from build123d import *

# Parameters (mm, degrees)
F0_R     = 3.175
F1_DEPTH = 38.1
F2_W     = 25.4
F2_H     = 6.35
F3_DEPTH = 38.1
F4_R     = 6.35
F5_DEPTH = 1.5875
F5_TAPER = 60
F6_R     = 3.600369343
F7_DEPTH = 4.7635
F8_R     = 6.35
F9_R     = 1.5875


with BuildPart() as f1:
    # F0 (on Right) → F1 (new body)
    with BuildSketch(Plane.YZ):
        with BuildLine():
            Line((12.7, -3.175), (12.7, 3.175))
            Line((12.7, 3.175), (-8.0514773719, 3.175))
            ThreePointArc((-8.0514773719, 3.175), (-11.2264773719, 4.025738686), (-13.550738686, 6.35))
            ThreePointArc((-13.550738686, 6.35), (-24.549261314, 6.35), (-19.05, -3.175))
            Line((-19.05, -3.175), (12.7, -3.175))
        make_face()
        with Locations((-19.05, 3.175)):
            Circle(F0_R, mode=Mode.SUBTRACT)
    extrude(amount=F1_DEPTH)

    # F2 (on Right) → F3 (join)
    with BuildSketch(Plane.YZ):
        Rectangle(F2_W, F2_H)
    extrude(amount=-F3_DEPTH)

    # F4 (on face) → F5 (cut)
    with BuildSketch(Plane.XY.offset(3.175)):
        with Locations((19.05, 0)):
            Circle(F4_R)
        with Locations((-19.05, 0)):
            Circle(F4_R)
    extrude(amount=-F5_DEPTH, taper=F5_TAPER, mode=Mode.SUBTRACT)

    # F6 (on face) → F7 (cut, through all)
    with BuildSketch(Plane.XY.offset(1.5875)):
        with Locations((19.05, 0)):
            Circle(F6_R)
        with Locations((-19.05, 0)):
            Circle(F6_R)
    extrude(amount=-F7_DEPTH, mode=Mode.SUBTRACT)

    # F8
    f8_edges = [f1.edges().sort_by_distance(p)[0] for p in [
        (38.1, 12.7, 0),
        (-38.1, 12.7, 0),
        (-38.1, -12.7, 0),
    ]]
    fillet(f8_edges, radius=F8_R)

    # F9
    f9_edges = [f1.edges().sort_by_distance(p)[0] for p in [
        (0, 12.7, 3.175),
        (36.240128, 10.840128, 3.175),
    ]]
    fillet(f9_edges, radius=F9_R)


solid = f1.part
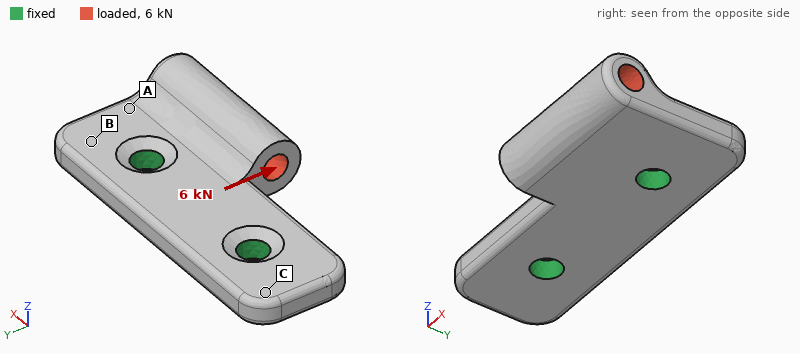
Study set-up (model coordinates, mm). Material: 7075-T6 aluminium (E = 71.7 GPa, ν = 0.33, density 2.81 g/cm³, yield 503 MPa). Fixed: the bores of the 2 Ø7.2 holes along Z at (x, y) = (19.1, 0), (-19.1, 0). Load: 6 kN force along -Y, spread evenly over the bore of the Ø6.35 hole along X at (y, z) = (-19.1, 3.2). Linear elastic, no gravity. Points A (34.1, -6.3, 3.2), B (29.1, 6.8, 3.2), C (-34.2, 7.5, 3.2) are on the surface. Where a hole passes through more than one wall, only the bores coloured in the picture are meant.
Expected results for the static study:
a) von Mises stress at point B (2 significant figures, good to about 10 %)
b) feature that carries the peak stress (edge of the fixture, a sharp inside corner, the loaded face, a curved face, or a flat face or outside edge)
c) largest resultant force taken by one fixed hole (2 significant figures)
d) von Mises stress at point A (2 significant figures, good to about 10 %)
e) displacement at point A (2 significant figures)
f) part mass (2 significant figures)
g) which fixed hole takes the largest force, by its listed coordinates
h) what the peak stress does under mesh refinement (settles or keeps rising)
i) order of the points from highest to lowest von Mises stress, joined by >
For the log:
26 MPa
edge of the fixture
5.8 kN
67 MPa
0.026 mm
43 g
(19.1, 0)
keeps rising
A > B > C
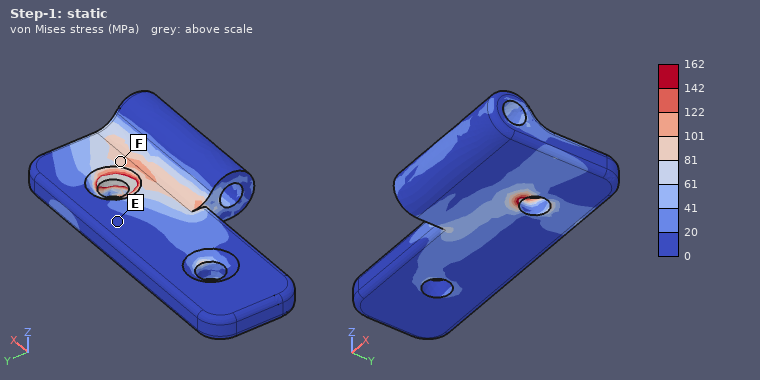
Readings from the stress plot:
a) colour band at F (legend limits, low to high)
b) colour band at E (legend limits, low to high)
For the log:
81 to 101 MPa
0 to 20 MPa
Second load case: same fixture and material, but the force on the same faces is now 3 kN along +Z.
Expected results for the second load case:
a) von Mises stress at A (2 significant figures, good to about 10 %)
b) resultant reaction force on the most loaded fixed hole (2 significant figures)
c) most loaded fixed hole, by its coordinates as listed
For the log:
93 MPa
2.9 kN
(19.1, 0)
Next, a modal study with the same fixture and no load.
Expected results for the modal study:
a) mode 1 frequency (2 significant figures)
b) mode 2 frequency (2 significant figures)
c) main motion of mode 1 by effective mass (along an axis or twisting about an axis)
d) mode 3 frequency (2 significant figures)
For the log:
6200 Hz
10 kHz
along Z
14 kHz
